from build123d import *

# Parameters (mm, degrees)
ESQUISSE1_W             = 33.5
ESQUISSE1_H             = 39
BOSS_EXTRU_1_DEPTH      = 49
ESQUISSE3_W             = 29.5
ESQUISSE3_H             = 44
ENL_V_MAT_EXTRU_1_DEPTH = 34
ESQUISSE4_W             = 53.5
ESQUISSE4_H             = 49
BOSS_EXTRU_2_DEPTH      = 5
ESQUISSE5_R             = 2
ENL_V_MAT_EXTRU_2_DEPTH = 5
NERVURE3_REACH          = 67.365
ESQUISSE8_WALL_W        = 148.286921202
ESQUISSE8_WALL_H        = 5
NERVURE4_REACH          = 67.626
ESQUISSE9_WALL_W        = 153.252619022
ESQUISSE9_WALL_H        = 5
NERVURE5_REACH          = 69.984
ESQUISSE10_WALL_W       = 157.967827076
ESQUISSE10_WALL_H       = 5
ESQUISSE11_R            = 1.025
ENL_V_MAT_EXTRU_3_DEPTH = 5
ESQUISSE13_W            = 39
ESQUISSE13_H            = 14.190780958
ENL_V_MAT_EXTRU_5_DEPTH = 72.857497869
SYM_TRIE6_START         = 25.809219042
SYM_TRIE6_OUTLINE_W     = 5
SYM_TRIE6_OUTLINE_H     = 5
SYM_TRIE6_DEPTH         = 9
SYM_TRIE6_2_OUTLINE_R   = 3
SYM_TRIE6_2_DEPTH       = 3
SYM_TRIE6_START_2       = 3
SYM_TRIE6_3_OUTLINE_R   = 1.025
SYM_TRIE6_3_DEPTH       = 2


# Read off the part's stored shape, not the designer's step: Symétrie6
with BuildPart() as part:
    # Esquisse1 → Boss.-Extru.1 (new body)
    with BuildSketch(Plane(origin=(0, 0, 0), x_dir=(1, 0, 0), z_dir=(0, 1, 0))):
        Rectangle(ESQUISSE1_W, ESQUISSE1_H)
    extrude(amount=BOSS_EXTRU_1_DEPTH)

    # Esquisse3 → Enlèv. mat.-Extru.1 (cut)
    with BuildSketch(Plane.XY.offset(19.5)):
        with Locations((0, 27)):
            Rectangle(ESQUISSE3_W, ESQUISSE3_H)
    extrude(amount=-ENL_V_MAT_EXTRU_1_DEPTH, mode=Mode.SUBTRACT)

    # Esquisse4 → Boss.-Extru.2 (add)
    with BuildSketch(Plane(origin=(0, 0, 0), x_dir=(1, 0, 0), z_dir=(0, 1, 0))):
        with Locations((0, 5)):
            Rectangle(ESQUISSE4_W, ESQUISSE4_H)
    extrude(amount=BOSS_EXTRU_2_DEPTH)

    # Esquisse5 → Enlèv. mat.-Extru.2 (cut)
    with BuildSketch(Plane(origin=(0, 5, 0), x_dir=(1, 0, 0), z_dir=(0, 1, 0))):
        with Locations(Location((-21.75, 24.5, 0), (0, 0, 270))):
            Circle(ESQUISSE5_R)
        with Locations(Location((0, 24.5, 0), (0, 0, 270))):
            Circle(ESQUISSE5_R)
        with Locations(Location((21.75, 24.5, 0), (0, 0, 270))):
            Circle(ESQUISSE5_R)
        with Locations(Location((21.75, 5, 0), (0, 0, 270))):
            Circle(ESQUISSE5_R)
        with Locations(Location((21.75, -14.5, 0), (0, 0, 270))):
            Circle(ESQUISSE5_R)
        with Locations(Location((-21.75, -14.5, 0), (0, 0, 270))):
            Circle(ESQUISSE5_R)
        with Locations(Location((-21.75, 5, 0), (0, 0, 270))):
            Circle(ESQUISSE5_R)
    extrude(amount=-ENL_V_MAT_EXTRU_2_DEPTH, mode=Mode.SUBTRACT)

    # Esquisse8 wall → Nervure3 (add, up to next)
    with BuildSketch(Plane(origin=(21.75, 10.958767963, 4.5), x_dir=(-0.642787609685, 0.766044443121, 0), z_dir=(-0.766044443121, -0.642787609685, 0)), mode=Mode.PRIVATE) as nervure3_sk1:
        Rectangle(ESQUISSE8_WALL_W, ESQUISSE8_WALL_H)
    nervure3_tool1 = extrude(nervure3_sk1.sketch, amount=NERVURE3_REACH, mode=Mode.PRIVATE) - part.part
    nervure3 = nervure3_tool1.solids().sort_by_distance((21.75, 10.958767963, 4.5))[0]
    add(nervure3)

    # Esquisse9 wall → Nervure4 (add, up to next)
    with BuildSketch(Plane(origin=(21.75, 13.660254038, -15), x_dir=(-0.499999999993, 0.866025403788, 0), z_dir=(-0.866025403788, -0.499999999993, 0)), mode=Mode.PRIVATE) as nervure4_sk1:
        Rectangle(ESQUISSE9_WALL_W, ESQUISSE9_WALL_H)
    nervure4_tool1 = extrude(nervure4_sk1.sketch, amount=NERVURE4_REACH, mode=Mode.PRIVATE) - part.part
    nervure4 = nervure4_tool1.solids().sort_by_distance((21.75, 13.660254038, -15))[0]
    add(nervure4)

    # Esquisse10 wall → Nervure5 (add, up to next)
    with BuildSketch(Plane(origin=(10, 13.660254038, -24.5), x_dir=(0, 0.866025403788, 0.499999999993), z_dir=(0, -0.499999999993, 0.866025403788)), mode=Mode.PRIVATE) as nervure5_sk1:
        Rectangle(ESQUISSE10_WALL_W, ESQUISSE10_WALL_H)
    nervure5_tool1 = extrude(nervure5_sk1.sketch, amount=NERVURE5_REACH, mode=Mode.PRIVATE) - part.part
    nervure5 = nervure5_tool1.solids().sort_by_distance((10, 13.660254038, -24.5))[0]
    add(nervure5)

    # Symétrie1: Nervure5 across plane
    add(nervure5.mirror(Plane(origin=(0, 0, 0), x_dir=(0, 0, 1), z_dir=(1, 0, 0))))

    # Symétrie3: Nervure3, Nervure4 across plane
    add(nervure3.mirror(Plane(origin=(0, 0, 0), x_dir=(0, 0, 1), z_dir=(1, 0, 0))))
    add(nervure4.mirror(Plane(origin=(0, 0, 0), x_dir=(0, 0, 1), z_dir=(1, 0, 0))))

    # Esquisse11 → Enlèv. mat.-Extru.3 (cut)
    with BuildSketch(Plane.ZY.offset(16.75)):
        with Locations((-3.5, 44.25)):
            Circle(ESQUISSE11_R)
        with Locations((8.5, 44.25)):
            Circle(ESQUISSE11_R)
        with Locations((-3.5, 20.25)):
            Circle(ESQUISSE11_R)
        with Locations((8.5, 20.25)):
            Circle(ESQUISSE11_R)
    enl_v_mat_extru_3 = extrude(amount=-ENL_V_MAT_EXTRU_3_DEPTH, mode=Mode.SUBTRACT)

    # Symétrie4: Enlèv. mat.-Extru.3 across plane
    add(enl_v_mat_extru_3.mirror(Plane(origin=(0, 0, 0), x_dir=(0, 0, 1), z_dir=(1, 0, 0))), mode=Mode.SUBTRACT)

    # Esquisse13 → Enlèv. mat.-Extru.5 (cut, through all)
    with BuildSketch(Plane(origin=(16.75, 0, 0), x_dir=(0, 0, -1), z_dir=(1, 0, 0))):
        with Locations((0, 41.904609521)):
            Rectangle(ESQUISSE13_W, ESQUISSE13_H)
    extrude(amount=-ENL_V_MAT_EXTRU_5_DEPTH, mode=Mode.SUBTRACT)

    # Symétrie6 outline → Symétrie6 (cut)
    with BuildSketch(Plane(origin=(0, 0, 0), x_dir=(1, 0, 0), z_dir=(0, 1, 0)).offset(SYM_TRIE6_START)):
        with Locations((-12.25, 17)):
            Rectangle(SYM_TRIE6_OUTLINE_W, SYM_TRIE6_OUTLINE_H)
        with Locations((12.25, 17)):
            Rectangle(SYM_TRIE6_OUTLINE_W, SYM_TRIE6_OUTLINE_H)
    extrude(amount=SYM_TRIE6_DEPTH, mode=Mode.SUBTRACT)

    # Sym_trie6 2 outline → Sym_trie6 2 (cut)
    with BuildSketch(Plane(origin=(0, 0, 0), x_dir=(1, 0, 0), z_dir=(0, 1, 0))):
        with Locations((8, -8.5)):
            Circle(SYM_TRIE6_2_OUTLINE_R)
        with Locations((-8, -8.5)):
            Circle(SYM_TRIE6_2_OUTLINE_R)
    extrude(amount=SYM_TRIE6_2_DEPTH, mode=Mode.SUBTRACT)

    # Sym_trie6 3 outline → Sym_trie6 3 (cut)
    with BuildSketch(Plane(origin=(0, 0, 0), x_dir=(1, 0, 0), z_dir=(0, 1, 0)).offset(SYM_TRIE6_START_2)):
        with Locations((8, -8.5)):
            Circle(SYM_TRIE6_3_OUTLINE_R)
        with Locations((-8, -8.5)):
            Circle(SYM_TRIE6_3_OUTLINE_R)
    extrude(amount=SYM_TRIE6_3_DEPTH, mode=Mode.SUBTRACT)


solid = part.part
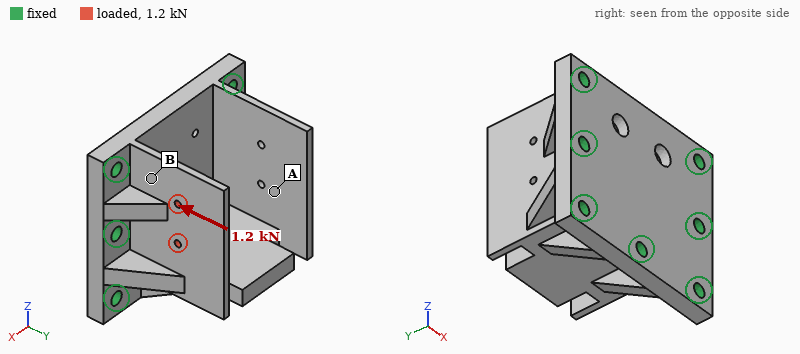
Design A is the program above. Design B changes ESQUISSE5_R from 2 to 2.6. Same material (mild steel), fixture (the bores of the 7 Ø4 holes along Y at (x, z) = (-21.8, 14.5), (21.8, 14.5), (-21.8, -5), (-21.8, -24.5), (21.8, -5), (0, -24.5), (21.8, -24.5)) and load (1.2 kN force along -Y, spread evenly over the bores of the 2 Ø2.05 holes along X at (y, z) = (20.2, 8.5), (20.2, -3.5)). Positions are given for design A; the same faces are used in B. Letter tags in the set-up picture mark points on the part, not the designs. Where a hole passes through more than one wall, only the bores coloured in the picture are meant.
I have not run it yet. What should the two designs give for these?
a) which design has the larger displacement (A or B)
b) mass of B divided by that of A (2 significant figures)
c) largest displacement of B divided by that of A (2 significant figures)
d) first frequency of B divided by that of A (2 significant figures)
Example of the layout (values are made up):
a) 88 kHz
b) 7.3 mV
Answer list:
a) A
b) 0.99
c) 0.90
d) 1.0
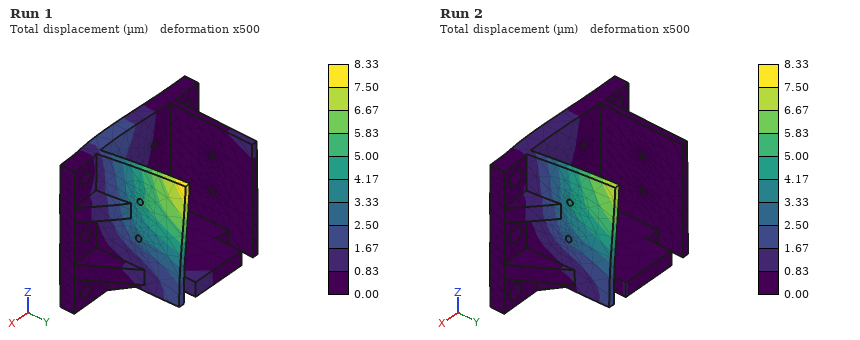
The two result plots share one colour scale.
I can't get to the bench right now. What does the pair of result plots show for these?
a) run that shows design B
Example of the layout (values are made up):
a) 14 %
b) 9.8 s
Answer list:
a) Run 2
